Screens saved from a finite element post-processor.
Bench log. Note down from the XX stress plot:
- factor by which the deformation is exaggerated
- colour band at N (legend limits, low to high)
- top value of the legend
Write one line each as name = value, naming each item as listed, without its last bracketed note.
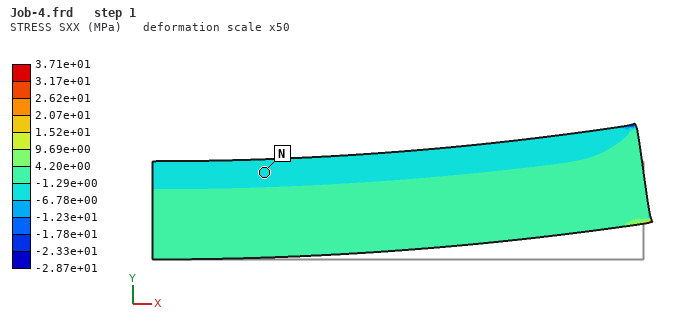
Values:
factor by which the deformation is exaggerated = 50
colour band at N = -6.78e+00 to -1.29e+00 MPa
top value of the legend = 3.71e+01 MPa
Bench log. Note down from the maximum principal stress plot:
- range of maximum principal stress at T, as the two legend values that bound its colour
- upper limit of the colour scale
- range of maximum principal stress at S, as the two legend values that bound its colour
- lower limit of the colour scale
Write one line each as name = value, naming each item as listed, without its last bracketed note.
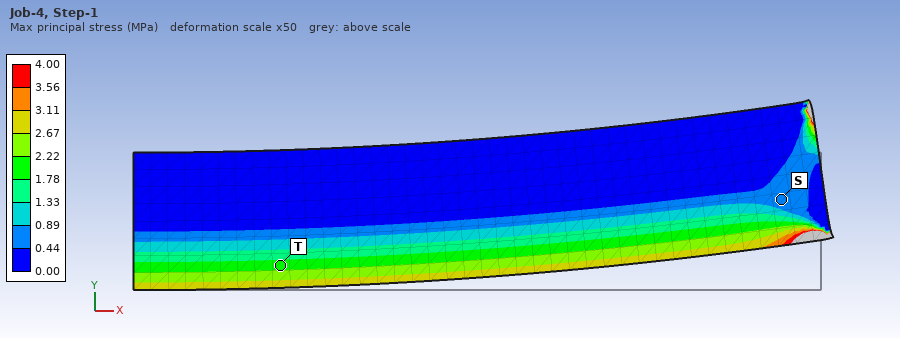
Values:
range of maximum principal stress at T, as the two legend values that bound its colour = 1.78 to 2.22 MPa
upper limit of the colour scale = 4.00 MPa
range of maximum principal stress at S, as the two legend values that bound its colour = 0.44 to 0.89 MPa
lower limit of the colour scale = 0.00 MPa
